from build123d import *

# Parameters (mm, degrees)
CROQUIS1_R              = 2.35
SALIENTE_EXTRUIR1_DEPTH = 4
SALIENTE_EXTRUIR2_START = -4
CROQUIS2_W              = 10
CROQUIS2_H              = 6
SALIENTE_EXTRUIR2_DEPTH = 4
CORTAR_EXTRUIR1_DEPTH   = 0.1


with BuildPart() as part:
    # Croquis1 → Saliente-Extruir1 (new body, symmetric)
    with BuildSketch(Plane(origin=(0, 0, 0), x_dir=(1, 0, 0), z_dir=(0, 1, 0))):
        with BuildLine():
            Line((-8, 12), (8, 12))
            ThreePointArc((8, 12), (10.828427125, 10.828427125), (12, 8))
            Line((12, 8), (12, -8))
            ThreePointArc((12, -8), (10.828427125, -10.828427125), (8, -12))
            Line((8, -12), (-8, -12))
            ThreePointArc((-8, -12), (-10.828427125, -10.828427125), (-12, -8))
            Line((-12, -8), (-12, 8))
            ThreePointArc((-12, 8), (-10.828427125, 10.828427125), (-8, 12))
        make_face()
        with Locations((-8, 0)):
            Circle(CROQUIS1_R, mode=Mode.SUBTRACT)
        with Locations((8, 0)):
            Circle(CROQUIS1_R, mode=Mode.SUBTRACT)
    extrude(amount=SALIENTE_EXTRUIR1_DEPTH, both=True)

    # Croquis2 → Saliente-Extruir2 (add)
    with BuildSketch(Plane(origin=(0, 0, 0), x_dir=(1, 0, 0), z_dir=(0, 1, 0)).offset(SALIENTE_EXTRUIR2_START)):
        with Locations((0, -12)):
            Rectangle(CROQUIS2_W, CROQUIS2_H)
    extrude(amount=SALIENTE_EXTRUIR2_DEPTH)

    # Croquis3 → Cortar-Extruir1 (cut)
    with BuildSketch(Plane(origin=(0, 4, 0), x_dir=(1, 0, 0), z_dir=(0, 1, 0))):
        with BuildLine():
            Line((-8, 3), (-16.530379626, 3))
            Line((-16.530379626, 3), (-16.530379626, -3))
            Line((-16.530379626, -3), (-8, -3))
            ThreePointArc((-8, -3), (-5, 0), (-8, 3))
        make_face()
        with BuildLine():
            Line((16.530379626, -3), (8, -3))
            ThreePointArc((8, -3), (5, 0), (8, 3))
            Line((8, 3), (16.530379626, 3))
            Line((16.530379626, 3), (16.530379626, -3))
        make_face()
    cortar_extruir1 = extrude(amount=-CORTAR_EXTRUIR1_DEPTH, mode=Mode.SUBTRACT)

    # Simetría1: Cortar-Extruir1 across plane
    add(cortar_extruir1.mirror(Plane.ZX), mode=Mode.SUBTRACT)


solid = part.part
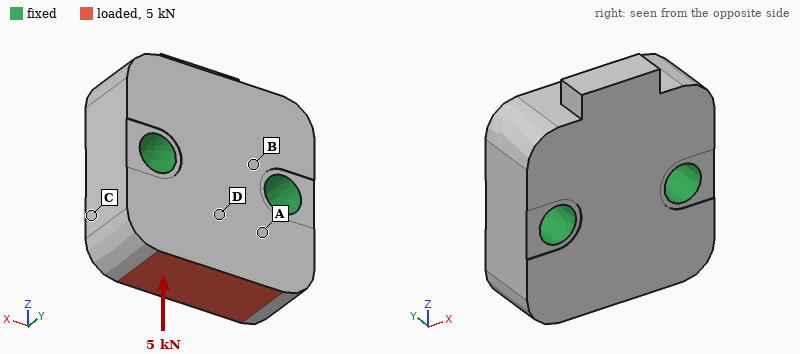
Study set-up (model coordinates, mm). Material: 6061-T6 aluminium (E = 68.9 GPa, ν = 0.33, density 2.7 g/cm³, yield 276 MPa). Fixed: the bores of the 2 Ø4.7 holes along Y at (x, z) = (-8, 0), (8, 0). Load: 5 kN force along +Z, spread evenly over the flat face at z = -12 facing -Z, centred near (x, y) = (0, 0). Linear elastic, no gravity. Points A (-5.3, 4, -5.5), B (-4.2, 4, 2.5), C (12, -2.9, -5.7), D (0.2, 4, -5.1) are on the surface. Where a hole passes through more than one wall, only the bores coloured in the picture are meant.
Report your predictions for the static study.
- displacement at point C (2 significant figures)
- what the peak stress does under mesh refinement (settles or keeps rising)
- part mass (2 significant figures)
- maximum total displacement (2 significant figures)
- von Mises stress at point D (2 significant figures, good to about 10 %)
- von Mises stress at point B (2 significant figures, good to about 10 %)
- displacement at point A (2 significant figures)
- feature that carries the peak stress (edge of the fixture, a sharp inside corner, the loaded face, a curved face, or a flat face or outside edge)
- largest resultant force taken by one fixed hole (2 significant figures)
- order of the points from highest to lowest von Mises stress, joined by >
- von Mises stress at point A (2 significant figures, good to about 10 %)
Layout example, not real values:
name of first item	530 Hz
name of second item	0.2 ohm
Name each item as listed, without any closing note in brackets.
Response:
displacement at point C	1.5 µm
what the peak stress does under mesh refinement	keeps rising
part mass	12 g
maximum total displacement	6.9 µm
von Mises stress at point D	26 MPa
von Mises stress at point B	16 MPa
displacement at point A	2.6 µm
feature that carries the peak stress	edge of the fixture
largest resultant force taken by one fixed hole	2.6 kN
order of the points from highest to lowest von Mises stress, joined by >	A > D > B > C
von Mises stress at point A	39 MPa
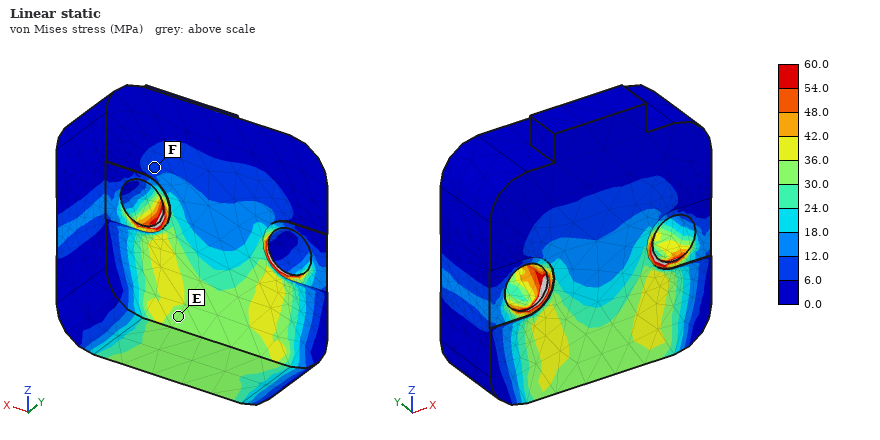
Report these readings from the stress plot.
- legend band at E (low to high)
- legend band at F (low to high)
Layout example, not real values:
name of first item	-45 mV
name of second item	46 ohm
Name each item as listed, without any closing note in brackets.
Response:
legend band at E	30.0 to 36.0 MPa
legend band at F	6.0 to 12.0 MPa
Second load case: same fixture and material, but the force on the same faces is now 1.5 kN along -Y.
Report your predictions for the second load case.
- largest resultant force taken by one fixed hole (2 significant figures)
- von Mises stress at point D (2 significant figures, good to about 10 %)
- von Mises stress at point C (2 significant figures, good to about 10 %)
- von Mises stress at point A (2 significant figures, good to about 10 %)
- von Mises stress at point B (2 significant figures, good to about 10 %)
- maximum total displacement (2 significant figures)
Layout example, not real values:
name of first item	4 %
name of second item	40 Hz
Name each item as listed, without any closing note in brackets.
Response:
largest resultant force taken by one fixed hole	750 N
von Mises stress at point D	34 MPa
von Mises stress at point C	18 MPa
von Mises stress at point A	44 MPa
von Mises stress at point B	17 MPa
maximum total displacement	19 µm
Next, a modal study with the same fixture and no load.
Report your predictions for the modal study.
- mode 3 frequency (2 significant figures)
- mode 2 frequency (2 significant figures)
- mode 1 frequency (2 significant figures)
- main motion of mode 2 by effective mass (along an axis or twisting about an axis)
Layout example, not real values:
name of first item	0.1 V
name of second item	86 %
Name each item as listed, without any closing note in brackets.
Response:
mode 3 frequency	56 kHz
mode 2 frequency	40 kHz
mode 1 frequency	34 kHz
main motion of mode 2 by effective mass	along Y
